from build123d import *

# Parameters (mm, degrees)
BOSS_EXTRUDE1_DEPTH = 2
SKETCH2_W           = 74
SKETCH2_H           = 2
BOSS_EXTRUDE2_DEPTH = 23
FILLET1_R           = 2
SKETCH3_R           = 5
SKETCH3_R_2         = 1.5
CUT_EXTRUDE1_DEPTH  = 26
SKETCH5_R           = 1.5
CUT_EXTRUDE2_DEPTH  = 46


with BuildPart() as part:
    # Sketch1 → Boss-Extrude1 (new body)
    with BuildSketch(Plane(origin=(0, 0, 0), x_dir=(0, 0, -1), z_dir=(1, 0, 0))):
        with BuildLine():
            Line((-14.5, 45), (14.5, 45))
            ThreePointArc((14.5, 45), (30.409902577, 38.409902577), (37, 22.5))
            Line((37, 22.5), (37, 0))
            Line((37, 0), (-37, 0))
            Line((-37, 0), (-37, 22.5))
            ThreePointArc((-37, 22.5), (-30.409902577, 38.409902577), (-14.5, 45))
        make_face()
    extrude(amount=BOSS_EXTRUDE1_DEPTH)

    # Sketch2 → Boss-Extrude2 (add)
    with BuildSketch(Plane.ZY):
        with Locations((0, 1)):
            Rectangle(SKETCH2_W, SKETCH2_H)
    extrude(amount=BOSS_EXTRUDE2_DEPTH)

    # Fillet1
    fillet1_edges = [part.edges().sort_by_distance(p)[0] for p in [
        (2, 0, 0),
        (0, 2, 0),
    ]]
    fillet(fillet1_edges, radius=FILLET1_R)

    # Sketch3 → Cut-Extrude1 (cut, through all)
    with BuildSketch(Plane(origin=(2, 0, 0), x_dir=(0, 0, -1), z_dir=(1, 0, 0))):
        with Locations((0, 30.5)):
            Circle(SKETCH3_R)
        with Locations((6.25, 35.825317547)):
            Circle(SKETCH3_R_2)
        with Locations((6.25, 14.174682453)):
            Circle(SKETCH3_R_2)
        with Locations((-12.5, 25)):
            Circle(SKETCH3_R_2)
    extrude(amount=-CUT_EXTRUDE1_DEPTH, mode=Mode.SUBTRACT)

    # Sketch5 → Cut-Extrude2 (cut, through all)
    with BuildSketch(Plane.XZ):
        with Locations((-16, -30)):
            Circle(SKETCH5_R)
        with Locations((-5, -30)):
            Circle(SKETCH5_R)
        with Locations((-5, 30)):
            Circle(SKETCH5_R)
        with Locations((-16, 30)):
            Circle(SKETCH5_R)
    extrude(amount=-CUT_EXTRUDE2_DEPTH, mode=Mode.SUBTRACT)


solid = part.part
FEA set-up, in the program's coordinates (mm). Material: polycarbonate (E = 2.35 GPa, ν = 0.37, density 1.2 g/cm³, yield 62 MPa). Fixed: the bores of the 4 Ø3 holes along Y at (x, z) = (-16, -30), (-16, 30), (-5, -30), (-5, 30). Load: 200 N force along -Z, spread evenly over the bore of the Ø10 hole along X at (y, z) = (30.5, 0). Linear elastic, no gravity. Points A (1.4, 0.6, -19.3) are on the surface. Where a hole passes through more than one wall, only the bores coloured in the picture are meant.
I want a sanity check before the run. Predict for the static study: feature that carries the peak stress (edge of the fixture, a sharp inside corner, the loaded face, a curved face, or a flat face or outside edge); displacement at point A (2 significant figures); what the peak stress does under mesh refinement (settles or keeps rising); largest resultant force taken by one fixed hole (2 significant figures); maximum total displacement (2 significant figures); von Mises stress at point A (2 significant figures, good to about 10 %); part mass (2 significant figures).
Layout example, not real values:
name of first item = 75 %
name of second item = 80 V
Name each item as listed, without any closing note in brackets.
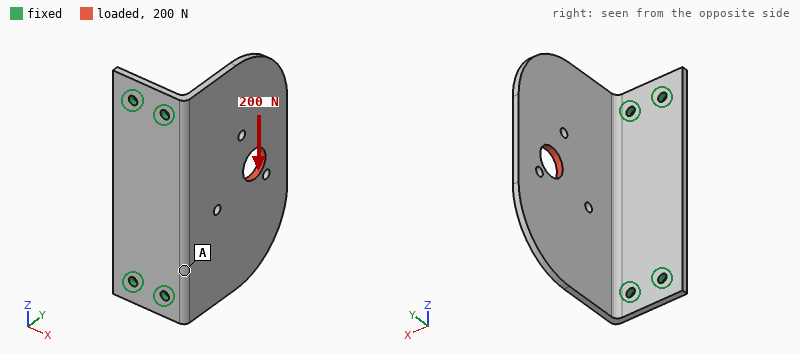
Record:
feature that carries the peak stress = edge of the fixture
displacement at point A = 0.14 mm
what the peak stress does under mesh refinement = keeps rising
largest resultant force taken by one fixed hole = 130 N
maximum total displacement = 0.89 mm
von Mises stress at point A = 3.5 MPa
part mass = 11 g
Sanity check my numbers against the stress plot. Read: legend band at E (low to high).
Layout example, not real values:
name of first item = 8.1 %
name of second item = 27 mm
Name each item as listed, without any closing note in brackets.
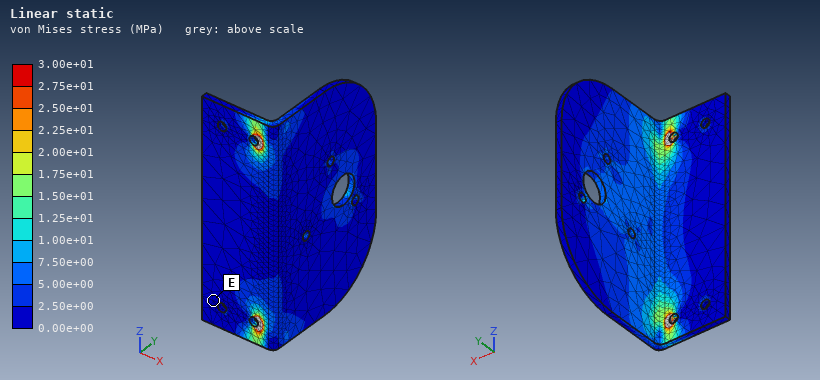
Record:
legend band at E = 0.00e+00 to 2.50e+00 MPa
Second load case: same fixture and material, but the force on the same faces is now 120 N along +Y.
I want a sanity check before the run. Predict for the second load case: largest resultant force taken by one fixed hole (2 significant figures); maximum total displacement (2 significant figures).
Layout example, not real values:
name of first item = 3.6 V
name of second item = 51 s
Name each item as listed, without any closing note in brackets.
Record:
largest resultant force taken by one fixed hole = 75 N
maximum total displacement = 1.1 mm
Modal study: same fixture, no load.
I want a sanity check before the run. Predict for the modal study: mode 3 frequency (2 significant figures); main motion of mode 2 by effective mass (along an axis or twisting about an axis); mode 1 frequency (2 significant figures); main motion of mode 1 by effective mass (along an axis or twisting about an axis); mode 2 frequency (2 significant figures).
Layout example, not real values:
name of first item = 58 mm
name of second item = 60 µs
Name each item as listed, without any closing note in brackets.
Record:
mode 3 frequency = 940 Hz
main motion of mode 2 by effective mass = twisting about Y
mode 1 frequency = 220 Hz
main motion of mode 1 by effective mass = along X
mode 2 frequency = 450 Hz
